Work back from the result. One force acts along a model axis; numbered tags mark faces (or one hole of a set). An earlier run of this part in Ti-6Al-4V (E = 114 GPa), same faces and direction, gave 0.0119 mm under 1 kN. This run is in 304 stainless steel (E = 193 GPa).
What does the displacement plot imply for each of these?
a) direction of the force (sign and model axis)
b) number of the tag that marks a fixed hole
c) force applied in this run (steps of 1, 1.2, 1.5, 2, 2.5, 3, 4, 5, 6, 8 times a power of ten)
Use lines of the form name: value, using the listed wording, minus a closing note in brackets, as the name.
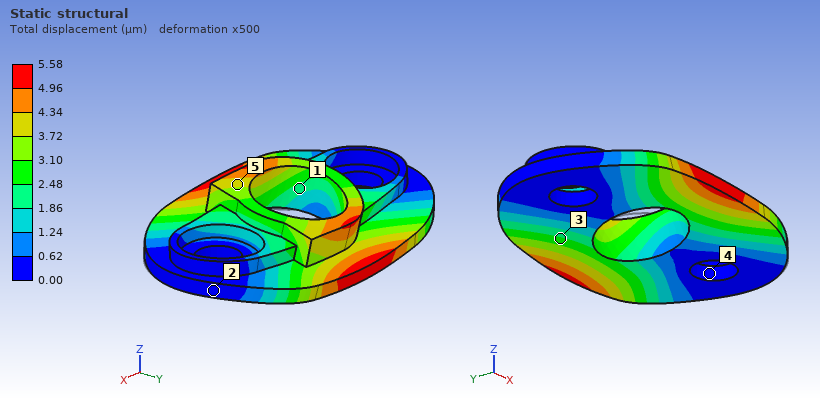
direction of the force: +Y
number of the tag that marks a fixed hole: 4
force applied in this run: 800 N
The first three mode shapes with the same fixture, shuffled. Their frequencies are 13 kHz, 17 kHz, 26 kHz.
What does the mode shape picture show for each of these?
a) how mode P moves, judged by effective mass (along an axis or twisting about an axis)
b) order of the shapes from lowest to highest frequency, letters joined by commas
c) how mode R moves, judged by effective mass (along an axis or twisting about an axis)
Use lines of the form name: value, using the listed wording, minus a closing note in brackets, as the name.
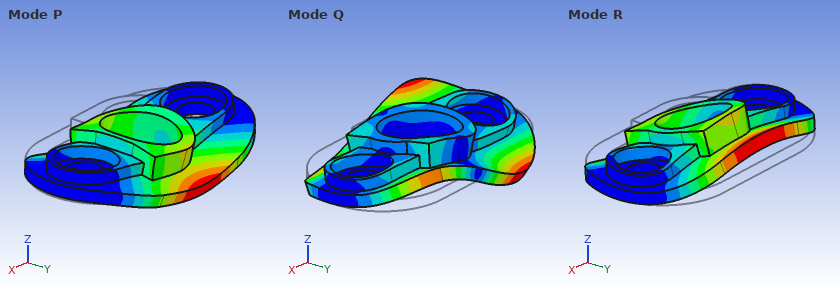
how mode P moves, judged by effective mass: along Z
order of the shapes from lowest to highest frequency, letters joined by commas: R, P, Q
how mode R moves, judged by effective mass: twisting about X
